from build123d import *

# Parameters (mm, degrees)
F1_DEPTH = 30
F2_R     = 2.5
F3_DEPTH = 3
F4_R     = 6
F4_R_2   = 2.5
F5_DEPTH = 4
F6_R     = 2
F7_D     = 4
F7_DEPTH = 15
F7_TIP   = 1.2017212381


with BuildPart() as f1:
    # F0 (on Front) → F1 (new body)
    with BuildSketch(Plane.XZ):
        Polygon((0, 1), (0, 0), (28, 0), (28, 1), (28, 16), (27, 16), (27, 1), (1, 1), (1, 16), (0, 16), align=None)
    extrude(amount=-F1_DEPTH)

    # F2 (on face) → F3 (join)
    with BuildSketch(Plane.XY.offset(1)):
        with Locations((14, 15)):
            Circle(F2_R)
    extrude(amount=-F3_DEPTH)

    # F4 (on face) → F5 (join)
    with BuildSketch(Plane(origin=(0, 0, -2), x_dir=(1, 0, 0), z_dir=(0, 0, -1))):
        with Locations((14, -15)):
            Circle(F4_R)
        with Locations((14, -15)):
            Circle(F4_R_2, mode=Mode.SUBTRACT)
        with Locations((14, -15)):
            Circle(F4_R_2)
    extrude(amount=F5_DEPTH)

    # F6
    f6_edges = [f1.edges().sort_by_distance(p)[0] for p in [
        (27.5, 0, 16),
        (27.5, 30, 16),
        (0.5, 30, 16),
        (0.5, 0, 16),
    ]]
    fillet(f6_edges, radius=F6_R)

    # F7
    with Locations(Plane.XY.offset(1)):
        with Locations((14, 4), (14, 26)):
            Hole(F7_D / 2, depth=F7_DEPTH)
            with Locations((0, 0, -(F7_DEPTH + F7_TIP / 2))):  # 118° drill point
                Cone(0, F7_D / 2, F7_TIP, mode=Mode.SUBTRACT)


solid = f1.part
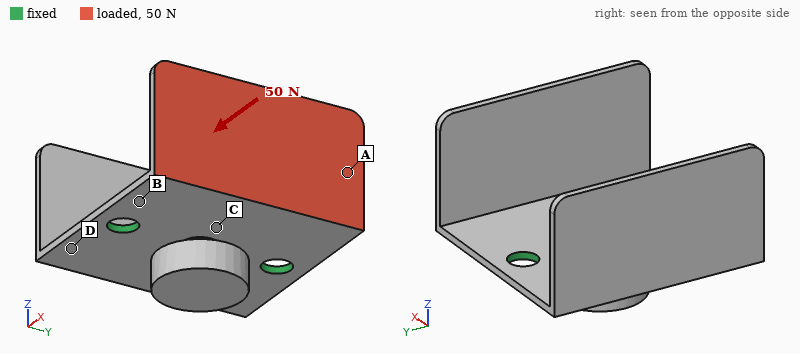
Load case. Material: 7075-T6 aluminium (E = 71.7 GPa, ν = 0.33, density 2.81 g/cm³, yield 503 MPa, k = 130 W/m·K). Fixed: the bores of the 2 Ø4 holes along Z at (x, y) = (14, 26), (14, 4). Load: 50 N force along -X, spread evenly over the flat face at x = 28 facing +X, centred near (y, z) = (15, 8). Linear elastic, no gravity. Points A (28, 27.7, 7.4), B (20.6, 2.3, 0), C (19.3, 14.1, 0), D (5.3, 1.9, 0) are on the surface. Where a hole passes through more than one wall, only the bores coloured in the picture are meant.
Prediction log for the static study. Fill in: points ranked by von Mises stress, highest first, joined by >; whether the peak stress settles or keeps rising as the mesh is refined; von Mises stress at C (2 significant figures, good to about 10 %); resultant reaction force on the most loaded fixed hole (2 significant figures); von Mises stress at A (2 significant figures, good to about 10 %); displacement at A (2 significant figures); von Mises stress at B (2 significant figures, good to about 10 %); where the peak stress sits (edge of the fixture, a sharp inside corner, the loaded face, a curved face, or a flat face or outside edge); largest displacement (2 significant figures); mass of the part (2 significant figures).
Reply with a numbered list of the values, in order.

1. B > C > A > D
2. keeps rising
3. 59 MPa
4. 26 N
5. 22 MPa
6. 0.26 mm
7. 73 MPa
8. edge of the fixture
9. 0.50 mm
10. 6.2 g
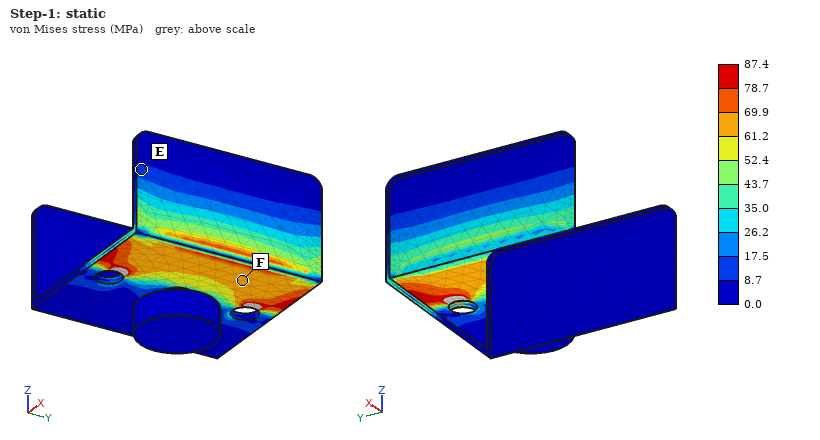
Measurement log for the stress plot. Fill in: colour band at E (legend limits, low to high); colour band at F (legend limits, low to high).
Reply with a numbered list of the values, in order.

1. 8.7 to 17.5 MPa
2. 61.2 to 69.9 MPa
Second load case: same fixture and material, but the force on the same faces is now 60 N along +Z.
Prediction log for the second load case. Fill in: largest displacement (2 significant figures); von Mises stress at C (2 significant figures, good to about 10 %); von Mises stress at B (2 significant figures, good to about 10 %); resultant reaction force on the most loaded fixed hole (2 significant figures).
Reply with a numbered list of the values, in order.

1. 0.49 mm
2. 77 MPa
3. 94 MPa
4. 31 N
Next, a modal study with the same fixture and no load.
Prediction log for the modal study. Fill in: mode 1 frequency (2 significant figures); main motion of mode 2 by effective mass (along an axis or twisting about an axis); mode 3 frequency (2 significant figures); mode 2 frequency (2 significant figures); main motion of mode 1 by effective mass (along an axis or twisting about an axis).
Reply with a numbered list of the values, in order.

1. 1400 Hz
2. along Z
3. 2700 Hz
4. 1500 Hz
5. along X
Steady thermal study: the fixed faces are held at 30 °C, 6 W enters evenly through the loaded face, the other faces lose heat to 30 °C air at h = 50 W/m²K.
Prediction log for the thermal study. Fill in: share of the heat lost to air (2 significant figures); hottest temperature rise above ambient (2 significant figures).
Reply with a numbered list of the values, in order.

1. 21 %
2. 28 K
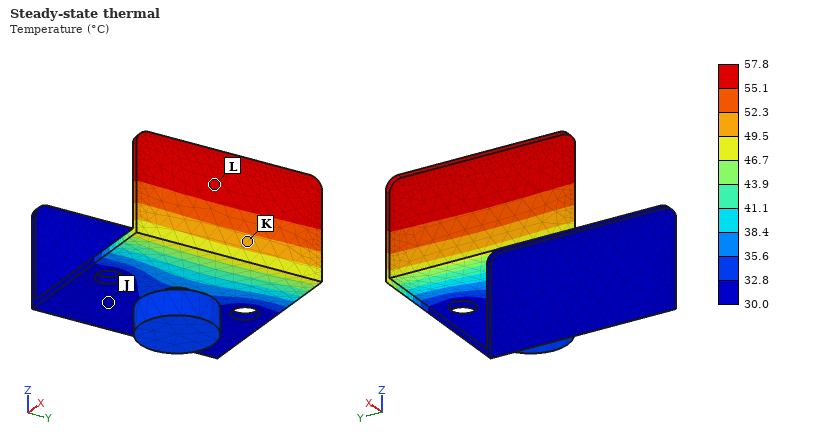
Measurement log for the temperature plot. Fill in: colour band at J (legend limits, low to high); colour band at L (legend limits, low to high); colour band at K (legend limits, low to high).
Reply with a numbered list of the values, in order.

1. 30.0 to 32.8 °C
2. 55.1 to 57.8 °C
3. 49.5 to 52.3 °C
